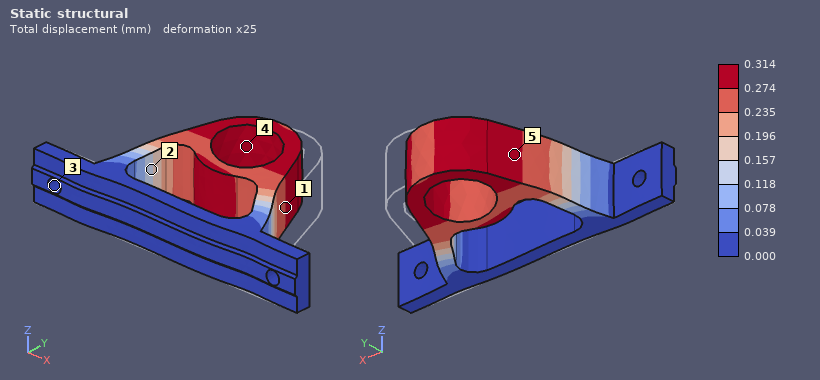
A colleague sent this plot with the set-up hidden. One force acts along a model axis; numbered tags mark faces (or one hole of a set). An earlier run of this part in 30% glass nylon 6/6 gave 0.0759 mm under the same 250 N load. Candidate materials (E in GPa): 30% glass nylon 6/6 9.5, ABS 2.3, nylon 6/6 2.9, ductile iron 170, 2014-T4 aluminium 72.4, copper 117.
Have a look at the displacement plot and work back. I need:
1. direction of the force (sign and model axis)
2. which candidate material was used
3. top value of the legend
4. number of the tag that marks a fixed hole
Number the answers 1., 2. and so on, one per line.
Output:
1. -X
2. ABS
3. 0.314 mm
4. 3
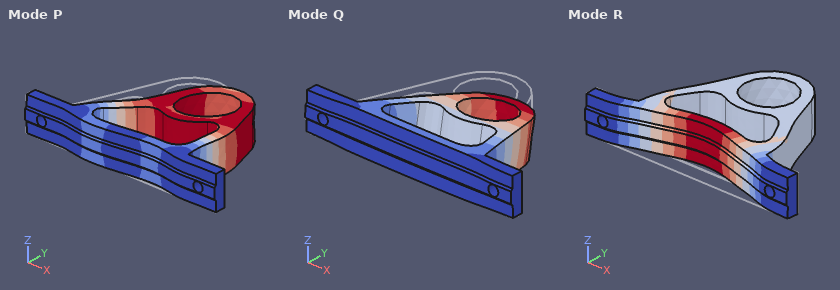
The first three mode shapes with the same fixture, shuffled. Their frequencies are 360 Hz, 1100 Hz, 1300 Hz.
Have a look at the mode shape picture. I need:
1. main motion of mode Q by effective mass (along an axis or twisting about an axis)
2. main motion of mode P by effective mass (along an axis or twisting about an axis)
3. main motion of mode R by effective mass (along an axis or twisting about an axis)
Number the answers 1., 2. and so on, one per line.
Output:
1. along Z
2. along X
3. along Y
